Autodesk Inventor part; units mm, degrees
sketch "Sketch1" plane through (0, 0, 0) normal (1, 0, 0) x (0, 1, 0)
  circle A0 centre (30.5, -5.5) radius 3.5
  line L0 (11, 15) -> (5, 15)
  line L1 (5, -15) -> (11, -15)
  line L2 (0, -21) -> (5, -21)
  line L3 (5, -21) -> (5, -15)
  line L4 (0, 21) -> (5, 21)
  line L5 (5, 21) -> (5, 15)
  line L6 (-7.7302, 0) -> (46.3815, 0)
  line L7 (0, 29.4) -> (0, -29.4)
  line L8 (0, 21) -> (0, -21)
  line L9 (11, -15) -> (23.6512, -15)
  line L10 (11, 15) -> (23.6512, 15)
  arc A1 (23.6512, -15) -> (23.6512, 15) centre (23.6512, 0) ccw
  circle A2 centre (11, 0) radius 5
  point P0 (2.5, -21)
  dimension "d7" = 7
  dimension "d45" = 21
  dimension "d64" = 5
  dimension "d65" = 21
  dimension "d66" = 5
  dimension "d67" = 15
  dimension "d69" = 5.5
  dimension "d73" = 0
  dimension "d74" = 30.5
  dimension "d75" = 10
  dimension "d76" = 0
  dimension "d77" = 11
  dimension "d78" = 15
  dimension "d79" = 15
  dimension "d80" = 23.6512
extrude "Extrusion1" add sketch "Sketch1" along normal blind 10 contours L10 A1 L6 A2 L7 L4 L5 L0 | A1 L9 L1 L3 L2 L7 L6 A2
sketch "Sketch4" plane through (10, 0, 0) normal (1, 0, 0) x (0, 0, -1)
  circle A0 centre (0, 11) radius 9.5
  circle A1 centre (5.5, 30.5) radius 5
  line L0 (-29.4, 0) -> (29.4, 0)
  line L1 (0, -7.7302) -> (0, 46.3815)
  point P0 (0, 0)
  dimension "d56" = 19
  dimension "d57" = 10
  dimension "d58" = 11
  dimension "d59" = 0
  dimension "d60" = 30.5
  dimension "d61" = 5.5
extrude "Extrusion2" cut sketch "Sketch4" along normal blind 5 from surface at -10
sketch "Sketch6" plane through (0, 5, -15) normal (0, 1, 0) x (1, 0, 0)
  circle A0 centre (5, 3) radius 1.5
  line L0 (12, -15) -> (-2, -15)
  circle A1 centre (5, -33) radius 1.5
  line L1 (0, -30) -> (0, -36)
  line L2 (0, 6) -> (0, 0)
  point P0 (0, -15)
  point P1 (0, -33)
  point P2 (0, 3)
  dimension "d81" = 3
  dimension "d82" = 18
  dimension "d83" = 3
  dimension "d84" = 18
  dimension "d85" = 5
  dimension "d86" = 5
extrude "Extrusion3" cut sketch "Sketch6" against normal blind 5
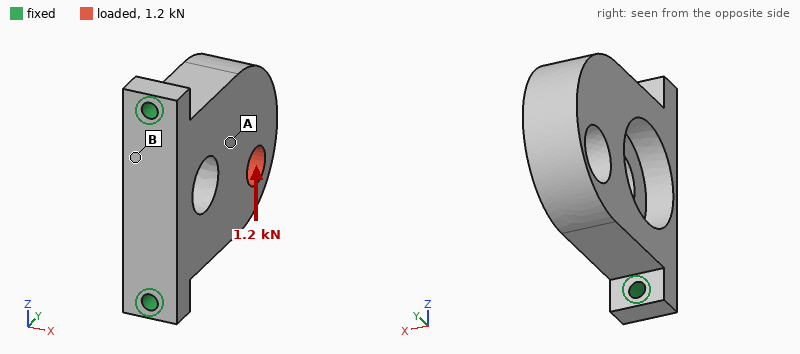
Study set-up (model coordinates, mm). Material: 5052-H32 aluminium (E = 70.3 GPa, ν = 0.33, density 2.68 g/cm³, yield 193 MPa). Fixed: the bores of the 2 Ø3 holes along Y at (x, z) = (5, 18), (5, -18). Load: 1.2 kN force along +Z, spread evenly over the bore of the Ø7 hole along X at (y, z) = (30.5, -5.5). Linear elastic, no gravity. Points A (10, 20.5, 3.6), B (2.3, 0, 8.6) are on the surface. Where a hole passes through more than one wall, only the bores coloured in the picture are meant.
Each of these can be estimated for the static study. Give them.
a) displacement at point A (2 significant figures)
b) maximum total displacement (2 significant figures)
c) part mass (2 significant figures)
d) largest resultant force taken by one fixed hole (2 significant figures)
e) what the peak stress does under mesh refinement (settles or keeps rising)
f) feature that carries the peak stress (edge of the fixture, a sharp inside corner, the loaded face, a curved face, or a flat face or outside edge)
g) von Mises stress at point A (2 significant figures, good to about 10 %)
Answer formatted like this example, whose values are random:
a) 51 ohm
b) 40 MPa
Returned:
a) 15 µm
b) 30 µm
c) 23 g
d) 1.2 kN
e) keeps rising
f) edge of the fixture
g) 18 MPa
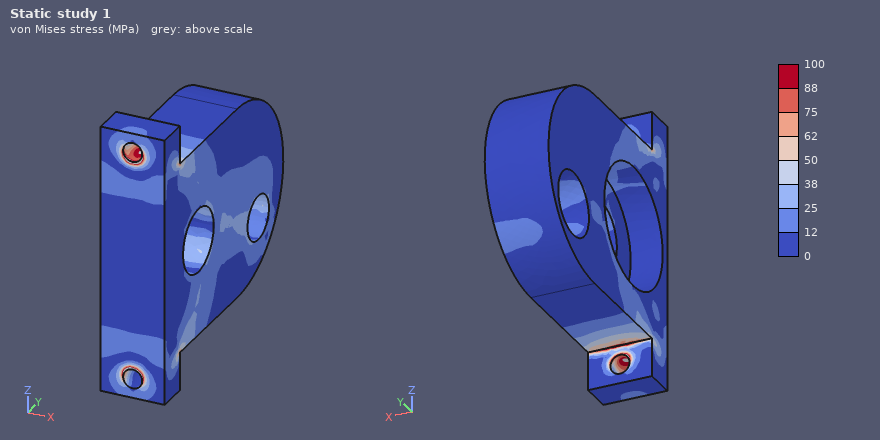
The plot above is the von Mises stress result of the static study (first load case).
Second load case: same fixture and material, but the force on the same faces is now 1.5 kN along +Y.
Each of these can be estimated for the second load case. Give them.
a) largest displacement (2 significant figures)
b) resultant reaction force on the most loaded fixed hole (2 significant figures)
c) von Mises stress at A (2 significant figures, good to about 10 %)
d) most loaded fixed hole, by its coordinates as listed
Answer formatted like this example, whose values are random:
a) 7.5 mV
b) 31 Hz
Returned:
a) 57 µm
b) 1.0 kN
c) 13 MPa
d) (5, -18)
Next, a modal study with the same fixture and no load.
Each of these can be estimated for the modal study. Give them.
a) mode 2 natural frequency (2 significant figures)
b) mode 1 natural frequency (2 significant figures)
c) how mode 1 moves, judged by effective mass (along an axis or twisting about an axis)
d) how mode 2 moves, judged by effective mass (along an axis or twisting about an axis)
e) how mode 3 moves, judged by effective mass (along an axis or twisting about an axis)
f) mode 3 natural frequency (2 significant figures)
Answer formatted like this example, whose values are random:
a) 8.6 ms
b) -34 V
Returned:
a) 10 kHz
b) 2900 Hz
c) along X
d) along Z
e) along Z
f) 12 kHz
